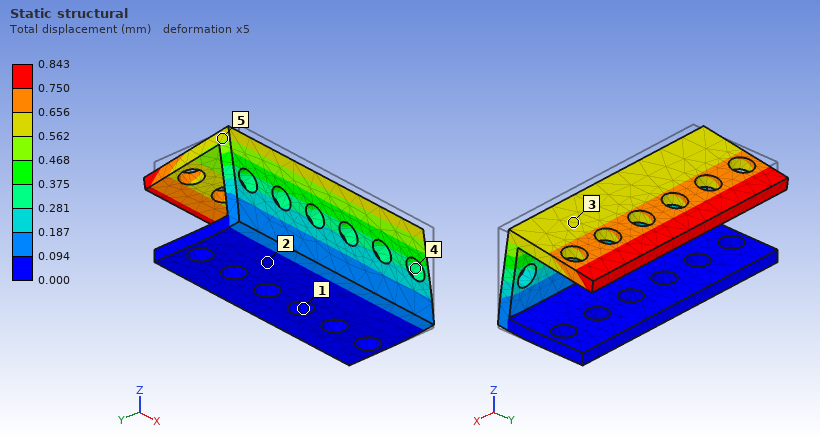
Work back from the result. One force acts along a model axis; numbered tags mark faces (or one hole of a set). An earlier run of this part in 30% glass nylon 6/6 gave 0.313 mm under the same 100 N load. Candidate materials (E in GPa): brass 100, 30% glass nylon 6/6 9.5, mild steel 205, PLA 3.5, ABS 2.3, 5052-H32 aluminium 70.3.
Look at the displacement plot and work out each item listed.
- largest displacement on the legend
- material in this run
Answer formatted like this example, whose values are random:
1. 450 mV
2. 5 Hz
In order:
1. 0.843 mm
2. PLA
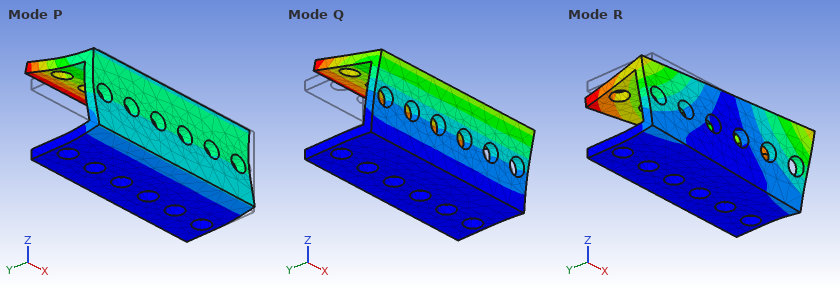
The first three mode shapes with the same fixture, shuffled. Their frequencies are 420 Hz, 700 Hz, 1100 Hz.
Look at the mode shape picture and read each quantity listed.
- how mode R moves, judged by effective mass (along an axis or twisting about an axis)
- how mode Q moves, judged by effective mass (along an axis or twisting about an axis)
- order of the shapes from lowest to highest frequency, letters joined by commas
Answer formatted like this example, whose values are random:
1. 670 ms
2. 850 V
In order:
1. along X
2. along Y
3. Q, R, P
